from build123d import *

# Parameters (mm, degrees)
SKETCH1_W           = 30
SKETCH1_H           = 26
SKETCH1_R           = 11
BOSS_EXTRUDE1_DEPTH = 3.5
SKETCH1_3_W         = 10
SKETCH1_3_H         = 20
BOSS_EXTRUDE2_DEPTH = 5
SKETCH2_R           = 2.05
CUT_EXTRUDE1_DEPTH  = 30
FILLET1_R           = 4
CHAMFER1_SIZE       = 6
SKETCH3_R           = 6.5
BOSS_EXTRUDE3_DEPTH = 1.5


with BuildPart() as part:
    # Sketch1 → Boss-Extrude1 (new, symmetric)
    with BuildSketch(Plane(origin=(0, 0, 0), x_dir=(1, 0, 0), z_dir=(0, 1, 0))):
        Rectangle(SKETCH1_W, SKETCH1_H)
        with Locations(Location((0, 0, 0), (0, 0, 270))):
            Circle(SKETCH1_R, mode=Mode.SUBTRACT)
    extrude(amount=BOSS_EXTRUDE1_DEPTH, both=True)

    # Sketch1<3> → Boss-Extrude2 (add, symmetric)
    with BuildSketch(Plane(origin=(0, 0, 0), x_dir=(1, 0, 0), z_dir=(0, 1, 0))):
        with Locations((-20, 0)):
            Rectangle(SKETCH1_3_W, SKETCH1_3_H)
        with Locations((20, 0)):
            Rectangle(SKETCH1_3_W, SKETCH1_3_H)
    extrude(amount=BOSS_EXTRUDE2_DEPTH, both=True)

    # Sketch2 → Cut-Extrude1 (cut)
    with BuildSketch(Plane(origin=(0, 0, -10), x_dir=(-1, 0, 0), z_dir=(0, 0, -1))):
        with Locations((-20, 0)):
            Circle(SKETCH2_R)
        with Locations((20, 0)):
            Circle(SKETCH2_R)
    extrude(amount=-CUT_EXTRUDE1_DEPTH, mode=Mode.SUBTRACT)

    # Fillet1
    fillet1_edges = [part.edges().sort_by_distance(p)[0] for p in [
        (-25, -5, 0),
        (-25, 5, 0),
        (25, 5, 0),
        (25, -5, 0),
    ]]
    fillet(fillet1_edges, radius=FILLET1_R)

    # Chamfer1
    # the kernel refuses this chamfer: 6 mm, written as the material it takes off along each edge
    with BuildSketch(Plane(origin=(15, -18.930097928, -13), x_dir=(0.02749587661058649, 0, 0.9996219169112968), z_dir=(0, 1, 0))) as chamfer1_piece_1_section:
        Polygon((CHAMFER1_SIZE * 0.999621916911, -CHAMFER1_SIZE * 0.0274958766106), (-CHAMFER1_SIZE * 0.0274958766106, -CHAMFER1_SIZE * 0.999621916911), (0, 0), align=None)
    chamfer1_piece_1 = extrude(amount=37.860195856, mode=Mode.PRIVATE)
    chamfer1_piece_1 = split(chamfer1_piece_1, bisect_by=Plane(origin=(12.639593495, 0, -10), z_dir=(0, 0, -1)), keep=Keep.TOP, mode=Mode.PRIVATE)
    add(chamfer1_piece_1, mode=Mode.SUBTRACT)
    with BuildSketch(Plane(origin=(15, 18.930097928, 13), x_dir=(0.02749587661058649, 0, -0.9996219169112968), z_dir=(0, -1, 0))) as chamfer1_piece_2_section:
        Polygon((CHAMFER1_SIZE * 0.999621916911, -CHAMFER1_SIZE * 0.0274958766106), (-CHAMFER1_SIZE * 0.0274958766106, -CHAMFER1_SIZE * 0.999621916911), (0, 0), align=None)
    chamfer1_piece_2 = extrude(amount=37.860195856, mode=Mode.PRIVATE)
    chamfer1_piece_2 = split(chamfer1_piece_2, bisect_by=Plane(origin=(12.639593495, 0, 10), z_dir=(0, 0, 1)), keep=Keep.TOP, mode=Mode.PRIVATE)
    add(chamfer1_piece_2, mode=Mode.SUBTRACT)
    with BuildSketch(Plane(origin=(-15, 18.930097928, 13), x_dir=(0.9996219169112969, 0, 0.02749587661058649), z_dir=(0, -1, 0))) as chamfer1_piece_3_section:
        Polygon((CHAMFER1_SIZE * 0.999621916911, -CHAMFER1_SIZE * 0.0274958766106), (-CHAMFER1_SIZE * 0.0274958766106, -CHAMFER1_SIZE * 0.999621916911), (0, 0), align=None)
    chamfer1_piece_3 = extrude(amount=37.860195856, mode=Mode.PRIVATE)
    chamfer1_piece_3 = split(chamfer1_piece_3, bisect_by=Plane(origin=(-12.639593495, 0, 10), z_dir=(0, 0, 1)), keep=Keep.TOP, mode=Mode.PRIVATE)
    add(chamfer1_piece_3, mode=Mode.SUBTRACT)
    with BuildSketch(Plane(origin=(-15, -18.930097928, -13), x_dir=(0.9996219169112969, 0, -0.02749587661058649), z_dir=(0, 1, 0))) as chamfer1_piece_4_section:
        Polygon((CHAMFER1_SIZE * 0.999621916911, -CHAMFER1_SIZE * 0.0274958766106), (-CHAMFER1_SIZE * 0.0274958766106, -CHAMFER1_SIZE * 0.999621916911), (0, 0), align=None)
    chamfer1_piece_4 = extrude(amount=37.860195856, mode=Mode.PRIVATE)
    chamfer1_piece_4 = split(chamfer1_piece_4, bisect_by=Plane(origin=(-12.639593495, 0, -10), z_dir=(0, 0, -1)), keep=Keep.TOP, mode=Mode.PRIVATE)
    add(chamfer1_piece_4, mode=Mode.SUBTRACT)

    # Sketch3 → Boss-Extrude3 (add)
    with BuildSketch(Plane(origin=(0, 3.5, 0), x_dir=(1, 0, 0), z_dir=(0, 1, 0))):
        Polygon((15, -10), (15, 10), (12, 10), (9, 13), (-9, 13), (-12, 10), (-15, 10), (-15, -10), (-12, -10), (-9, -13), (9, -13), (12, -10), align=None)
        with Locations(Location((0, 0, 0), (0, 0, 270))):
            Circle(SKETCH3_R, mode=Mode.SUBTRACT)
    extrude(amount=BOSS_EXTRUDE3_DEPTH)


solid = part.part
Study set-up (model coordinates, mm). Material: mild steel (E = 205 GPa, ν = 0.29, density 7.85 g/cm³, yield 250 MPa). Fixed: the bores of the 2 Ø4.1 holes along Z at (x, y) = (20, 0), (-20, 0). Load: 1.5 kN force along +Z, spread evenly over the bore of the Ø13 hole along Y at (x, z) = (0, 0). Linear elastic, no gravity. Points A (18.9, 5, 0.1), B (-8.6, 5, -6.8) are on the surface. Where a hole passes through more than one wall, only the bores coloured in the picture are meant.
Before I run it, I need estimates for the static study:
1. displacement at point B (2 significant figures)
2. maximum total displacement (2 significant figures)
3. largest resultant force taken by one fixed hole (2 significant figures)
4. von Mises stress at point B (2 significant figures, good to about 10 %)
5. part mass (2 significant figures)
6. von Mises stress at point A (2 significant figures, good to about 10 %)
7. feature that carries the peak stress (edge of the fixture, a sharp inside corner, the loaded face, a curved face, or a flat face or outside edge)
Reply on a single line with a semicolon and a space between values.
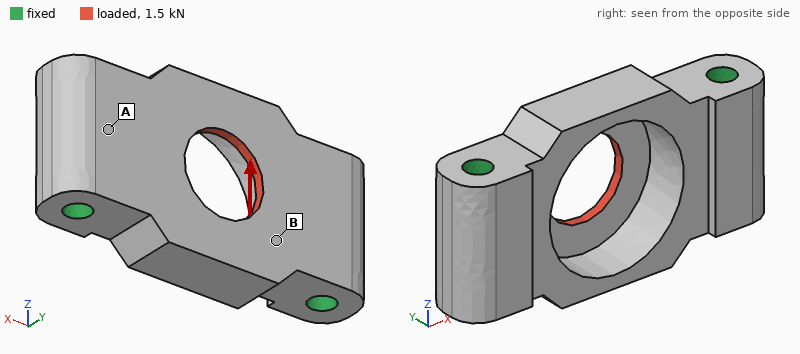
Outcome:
1.6 µm; 3.8 µm; 750 N; 27 MPa; 51 g; 6.8 MPa; a sharp inside corner
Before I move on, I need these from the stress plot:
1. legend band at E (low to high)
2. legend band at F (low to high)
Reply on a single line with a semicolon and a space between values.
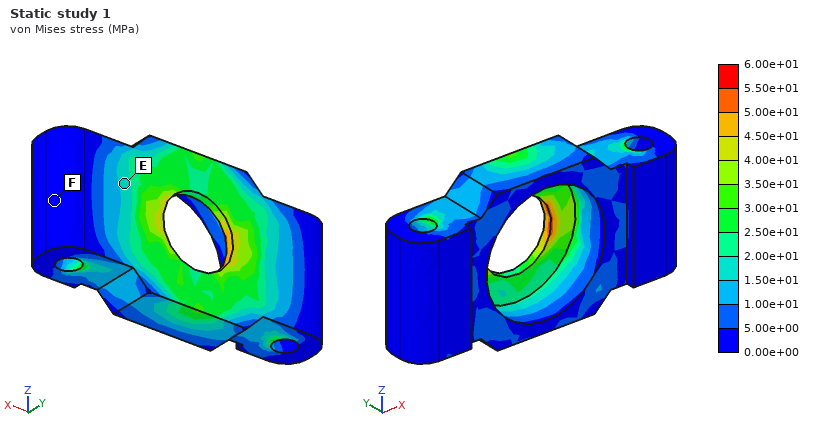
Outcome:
1.50e+01 to 2.00e+01 MPa; 0.00e+00 to 5.00e+00 MPa
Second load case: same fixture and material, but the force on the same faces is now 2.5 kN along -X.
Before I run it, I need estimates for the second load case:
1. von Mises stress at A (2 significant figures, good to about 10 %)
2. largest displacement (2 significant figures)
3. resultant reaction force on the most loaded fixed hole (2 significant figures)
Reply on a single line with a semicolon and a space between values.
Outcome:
7.8 MPa; 2.7 µm; 1.3 kN
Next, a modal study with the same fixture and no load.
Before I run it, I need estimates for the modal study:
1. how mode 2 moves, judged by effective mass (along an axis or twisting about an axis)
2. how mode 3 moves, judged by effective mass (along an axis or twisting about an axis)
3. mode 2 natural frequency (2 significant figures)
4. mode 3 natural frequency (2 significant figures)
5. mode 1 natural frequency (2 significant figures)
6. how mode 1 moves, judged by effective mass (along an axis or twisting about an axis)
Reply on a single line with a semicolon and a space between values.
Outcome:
twisting about X; along Z; 27 kHz; 43 kHz; 26 kHz; along Y
